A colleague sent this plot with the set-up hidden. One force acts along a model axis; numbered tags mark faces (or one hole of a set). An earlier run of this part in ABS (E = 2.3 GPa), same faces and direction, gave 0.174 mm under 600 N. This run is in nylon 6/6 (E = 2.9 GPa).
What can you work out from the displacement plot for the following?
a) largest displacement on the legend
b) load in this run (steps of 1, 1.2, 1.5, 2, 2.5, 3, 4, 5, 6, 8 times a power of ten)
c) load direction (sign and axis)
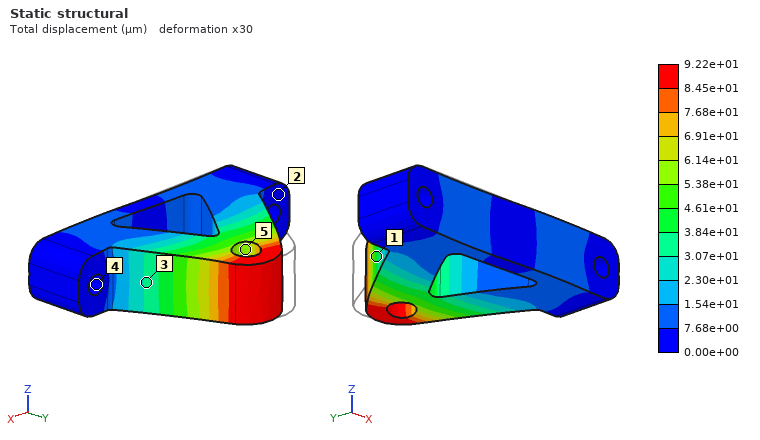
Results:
9.22e+01 µm
400 N
+X
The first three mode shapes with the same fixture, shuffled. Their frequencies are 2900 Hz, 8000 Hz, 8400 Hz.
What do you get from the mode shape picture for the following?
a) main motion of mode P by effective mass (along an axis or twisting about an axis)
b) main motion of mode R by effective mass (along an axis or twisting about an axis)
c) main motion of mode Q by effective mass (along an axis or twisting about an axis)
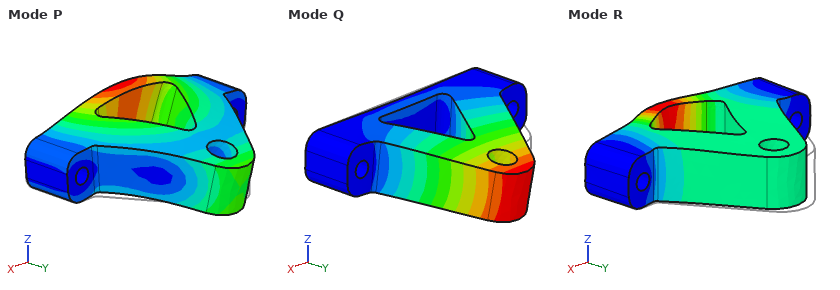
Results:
along Z
along Y
along Z
